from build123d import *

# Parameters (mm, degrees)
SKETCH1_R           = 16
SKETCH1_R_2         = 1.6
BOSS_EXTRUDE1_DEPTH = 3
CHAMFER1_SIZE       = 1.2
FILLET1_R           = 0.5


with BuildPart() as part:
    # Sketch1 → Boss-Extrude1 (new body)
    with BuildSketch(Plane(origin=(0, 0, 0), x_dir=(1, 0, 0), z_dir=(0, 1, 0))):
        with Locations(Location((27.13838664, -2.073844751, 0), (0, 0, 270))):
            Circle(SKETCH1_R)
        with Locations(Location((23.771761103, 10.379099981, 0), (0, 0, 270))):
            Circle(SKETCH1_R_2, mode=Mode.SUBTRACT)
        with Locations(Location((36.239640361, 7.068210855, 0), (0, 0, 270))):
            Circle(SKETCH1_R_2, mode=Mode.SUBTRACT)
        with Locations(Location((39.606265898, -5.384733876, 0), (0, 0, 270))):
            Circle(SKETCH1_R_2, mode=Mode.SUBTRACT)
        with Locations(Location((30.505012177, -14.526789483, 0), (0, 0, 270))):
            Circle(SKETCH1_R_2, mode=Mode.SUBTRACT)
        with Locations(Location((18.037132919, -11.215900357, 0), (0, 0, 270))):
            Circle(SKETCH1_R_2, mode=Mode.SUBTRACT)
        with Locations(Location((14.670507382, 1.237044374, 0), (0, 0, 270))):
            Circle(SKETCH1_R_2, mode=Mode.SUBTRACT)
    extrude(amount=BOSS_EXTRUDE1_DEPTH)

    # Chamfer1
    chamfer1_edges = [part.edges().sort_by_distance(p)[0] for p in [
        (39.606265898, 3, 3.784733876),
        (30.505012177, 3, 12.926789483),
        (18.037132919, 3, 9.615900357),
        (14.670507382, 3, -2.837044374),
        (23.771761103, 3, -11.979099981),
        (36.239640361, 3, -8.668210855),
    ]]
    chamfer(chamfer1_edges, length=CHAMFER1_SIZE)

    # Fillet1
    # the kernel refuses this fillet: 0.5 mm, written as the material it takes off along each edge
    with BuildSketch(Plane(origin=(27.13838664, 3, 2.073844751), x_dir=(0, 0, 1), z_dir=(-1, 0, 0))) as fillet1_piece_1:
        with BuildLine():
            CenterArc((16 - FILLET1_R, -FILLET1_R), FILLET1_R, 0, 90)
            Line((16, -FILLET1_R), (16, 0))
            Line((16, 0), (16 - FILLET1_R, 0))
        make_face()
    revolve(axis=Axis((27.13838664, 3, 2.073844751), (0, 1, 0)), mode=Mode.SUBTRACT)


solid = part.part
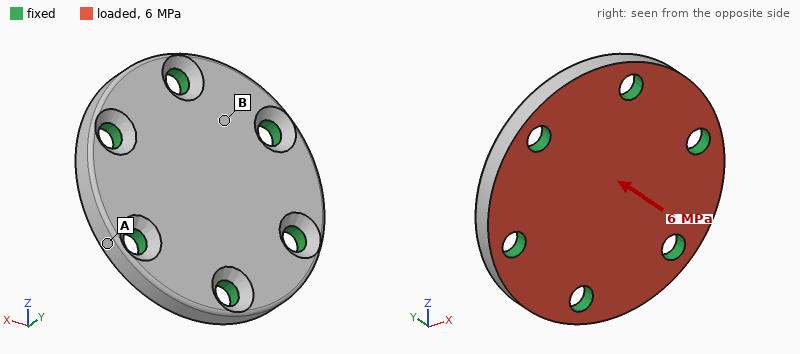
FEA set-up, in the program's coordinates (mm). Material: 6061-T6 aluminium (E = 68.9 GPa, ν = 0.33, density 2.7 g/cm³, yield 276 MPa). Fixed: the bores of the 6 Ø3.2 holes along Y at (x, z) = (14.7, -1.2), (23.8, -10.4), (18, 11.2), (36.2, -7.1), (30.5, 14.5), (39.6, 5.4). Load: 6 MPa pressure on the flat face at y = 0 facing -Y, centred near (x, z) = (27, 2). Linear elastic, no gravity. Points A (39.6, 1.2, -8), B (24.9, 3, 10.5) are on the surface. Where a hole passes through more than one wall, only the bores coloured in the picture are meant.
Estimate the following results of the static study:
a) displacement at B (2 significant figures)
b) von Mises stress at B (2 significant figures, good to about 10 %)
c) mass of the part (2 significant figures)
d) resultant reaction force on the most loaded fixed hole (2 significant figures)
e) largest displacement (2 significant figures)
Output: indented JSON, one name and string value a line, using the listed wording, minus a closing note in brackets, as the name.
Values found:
{
  "displacement at B": "9.9 µm",
  "von Mises stress at B": "48 MPa",
  "mass of the part": "6.0 g",
  "resultant reaction force on the most loaded fixed hole": "780 N",
  "largest displacement": "22 µm"
}
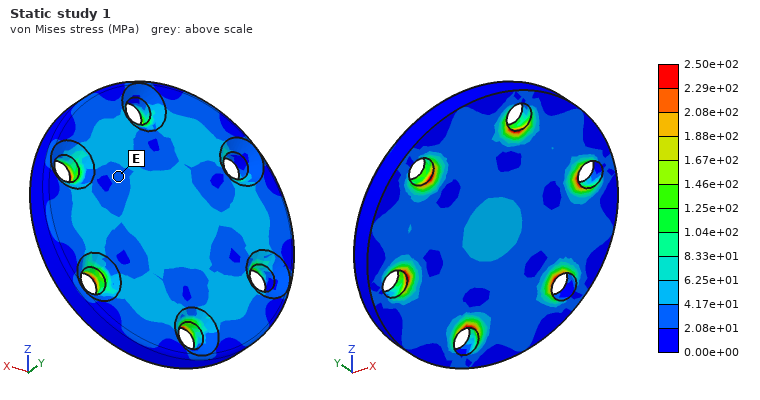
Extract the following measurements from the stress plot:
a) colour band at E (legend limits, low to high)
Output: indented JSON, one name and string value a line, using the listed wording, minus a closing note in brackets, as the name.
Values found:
{
  "colour band at E": "2.08e+01 to 4.17e+01 MPa"
}
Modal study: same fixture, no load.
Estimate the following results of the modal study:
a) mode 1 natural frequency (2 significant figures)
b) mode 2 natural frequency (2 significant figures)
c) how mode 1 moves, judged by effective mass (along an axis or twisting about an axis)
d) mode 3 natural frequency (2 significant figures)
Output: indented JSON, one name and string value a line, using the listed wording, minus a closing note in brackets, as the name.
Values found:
{
  "mode 1 natural frequency": "35 kHz",
  "mode 2 natural frequency": "63 kHz",
  "how mode 1 moves, judged by effective mass": "along Y",
  "mode 3 natural frequency": "64 kHz"
}
